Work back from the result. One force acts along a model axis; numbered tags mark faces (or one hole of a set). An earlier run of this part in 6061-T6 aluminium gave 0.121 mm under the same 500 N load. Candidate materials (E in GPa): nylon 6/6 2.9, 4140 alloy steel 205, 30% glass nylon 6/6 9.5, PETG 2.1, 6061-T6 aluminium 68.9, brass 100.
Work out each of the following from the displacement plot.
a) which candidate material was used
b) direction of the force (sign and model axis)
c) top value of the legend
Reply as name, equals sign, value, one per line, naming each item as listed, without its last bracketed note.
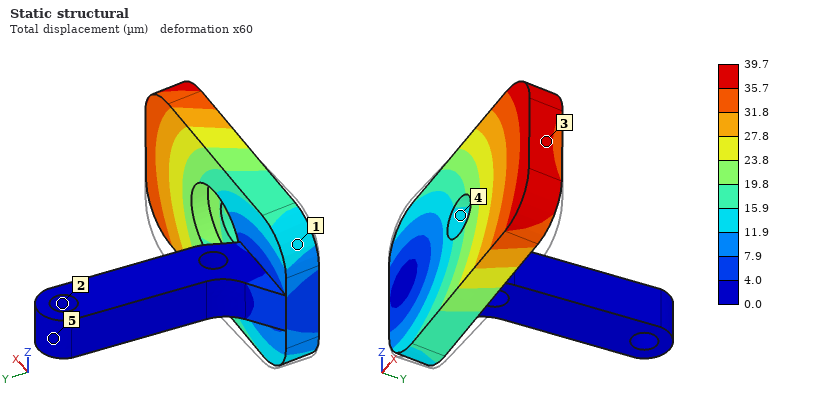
which candidate material was used = 4140 alloy steel
direction of the force = +Z
top value of the legend = 39.7 µm
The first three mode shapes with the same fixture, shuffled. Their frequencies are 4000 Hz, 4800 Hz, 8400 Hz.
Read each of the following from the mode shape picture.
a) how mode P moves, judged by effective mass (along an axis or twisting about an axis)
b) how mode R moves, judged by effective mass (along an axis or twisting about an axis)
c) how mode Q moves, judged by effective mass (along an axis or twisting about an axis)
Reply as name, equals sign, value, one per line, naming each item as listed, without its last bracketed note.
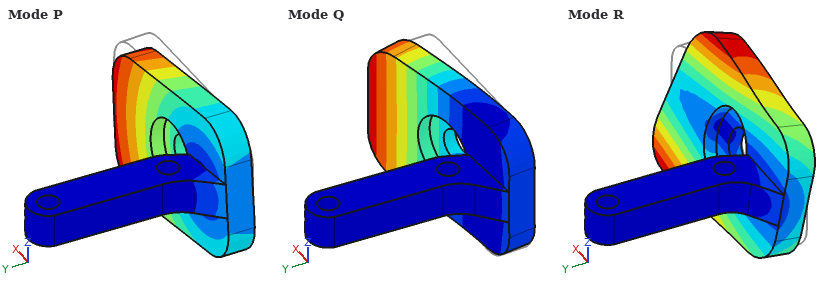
how mode P moves, judged by effective mass = along Z
how mode R moves, judged by effective mass = twisting about X
how mode Q moves, judged by effective mass = along Y
